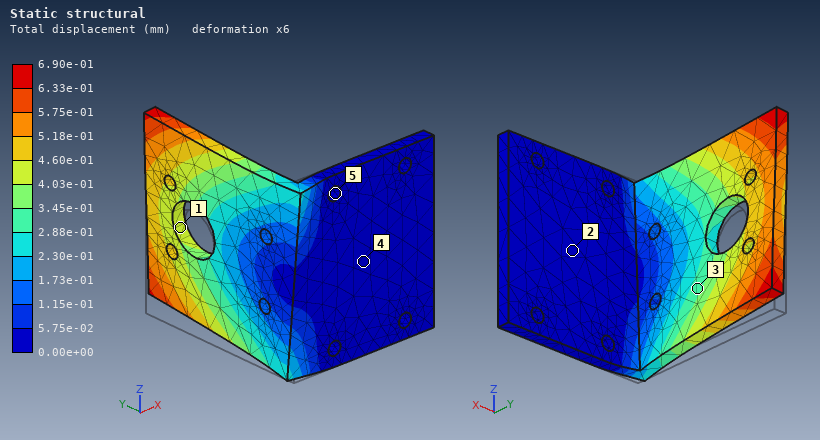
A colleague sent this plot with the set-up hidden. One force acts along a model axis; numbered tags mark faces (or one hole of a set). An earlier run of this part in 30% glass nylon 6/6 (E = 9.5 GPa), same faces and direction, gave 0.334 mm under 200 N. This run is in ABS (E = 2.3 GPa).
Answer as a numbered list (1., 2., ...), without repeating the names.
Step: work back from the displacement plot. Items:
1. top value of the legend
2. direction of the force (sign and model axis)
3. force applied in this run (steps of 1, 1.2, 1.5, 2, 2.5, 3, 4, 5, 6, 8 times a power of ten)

1. 6.90e-01 mm
2. +Z
3. 100 N
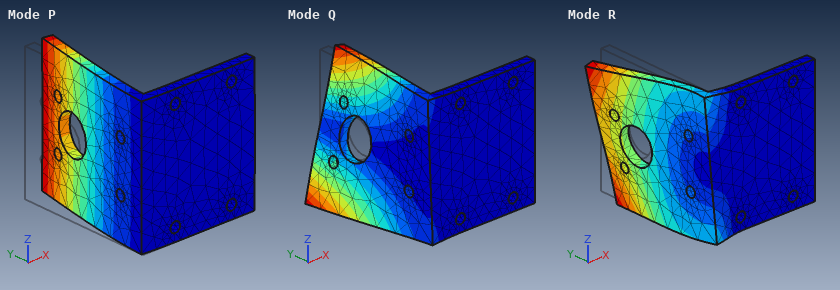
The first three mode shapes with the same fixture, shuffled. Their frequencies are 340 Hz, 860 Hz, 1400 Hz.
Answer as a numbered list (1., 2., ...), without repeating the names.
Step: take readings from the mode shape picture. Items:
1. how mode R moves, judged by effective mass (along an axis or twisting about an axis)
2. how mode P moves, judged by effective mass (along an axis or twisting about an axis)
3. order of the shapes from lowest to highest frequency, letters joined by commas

1. along Z
2. along X
3. P, Q, R
